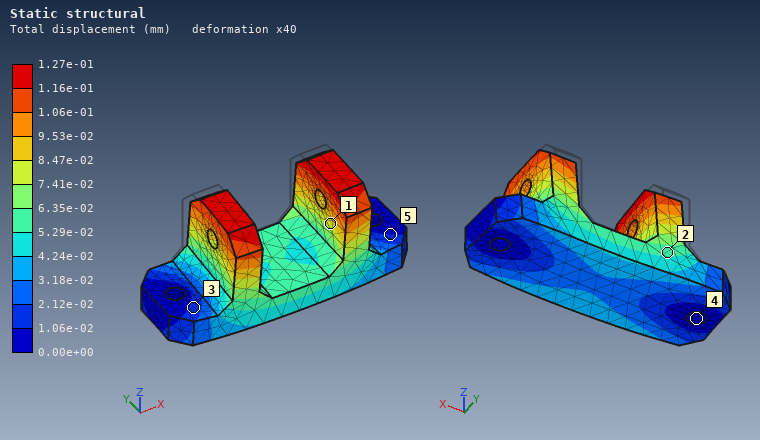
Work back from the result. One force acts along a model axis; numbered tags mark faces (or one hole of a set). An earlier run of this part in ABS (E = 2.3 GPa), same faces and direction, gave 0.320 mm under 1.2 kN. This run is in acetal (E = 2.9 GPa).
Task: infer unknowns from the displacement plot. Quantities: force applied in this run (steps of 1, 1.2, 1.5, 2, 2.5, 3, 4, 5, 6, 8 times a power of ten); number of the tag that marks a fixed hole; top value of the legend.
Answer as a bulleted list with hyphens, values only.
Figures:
- 600 N
- 4
- 1.27e-01 mm
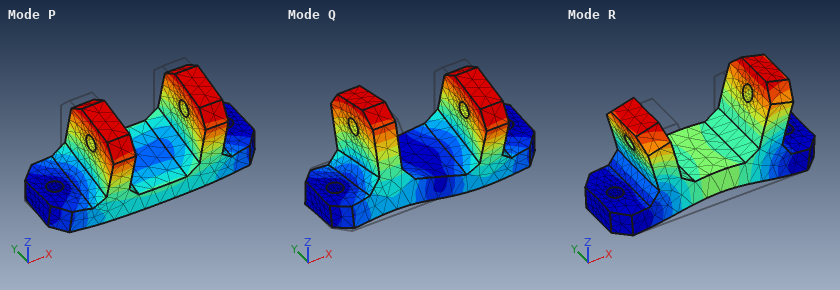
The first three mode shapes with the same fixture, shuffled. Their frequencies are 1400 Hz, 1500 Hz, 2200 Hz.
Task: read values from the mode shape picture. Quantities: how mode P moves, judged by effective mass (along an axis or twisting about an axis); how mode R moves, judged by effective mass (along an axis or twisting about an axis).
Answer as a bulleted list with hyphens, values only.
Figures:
- along Y
- along Z
